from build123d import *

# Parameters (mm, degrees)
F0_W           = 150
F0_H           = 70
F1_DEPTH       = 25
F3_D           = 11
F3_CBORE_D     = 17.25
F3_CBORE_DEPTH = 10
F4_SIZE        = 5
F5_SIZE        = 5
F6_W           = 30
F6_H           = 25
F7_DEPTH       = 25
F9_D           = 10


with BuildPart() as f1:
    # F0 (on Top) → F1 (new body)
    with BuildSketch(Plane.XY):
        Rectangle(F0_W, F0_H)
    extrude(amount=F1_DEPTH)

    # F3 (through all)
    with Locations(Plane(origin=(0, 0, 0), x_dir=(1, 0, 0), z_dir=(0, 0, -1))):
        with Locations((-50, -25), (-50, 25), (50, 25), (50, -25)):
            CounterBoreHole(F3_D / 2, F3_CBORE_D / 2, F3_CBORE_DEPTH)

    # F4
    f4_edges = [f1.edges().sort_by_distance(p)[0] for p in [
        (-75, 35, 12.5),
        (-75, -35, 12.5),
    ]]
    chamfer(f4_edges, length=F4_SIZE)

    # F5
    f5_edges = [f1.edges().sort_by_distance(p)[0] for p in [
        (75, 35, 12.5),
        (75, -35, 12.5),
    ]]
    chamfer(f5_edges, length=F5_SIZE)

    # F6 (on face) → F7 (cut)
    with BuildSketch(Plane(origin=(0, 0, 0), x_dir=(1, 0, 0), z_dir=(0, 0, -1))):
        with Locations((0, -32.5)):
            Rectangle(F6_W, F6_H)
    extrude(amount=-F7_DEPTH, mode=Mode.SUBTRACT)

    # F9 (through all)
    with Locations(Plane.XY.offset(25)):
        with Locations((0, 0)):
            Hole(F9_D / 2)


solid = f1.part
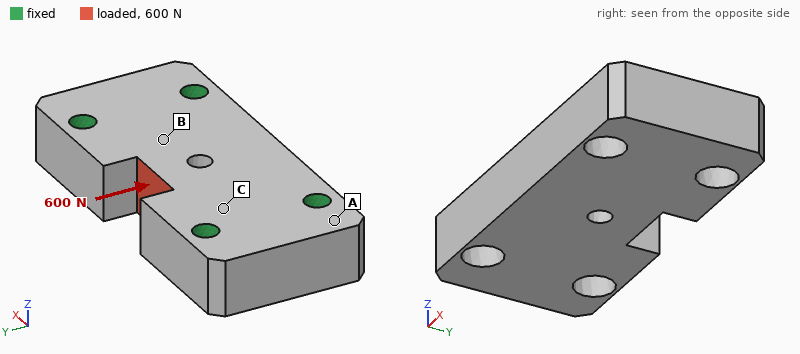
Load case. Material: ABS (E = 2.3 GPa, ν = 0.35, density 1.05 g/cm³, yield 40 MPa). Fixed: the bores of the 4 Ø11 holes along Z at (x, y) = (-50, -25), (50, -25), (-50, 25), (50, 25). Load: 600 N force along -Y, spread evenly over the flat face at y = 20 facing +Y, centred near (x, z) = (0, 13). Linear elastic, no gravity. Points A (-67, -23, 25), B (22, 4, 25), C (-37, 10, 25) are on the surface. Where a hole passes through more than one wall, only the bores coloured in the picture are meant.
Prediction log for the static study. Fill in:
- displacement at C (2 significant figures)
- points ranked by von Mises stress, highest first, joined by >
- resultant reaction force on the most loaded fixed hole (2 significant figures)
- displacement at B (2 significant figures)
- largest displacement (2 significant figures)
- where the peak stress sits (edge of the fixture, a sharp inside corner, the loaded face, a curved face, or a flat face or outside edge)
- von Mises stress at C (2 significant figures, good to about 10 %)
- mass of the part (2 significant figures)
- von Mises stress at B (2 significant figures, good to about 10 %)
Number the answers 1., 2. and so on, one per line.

1. 3.6 µm
2. B > C > A
3. 210 N
4. 9.3 µm
5. 21 µm
6. edge of the fixture
7. 0.42 MPa
8. 240 g
9. 0.54 MPa
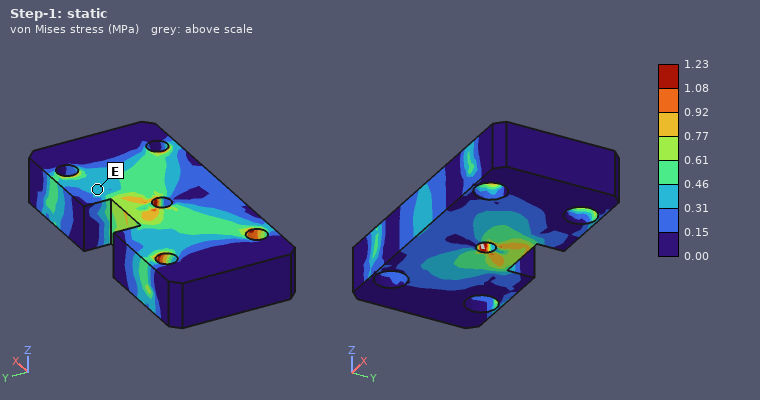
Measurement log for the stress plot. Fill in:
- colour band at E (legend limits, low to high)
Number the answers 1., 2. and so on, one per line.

1. 0.31 to 0.46 MPa
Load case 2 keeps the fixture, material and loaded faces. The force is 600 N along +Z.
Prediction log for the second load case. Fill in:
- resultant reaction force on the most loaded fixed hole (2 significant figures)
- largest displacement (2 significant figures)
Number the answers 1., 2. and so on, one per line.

1. 280 N
2. 85 µm
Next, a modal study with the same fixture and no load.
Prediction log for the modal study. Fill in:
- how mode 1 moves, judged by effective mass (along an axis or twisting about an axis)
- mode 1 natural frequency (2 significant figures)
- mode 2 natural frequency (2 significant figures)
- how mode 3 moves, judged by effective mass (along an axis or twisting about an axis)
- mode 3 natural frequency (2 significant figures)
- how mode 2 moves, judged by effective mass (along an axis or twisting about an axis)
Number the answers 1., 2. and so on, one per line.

1. along Z
2. 2300 Hz
3. 3600 Hz
4. along Y
5. 3800 Hz
6. twisting about X
